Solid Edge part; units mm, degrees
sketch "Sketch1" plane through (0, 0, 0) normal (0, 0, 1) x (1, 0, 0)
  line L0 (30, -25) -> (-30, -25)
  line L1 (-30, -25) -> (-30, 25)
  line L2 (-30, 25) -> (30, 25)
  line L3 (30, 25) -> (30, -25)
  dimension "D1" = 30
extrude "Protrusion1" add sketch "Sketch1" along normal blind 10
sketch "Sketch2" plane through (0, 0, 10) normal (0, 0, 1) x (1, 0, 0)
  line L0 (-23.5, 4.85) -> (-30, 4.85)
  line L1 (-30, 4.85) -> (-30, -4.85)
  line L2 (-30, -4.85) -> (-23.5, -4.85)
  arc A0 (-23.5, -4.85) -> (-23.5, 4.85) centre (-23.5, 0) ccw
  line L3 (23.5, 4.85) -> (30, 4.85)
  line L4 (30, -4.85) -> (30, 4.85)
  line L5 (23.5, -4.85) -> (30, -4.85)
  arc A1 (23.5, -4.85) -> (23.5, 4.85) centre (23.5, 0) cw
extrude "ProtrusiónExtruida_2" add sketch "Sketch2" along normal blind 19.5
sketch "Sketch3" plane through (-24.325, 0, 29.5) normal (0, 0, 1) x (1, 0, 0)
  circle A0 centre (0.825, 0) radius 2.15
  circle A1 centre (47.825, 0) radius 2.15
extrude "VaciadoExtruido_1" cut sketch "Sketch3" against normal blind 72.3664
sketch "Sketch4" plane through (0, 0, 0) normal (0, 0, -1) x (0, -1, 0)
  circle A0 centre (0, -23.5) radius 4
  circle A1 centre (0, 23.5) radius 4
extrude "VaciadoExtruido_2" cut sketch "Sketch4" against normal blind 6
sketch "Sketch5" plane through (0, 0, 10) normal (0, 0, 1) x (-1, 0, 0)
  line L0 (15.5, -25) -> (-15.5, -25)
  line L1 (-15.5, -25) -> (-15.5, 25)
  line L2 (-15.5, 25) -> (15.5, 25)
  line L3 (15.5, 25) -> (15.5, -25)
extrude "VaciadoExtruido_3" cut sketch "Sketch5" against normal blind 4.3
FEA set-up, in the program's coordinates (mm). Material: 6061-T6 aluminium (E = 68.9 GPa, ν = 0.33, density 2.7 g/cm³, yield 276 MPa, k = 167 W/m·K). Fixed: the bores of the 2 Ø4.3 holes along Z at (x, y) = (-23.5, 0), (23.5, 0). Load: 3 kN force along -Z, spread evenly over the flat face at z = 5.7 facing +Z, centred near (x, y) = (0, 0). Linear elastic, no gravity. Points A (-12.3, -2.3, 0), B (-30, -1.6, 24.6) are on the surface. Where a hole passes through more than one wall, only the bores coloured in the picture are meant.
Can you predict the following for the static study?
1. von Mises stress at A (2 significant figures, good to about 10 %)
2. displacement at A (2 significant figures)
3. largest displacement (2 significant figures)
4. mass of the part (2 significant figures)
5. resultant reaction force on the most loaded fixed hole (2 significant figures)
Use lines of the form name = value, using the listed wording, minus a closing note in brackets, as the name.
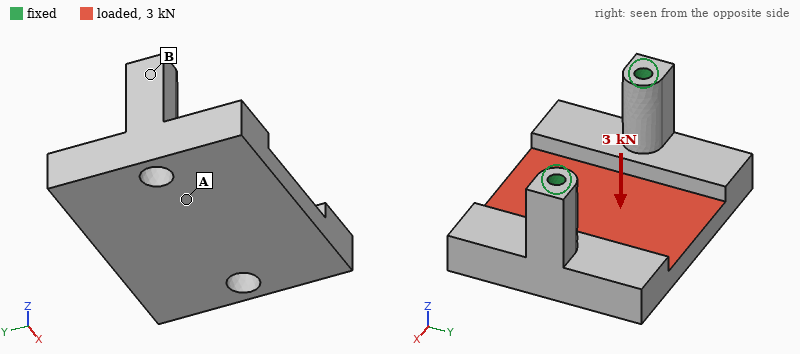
von Mises stress at A = 25 MPa
displacement at A = 13 µm
largest displacement = 39 µm
mass of the part = 70 g
resultant reaction force on the most loaded fixed hole = 2.2 kN
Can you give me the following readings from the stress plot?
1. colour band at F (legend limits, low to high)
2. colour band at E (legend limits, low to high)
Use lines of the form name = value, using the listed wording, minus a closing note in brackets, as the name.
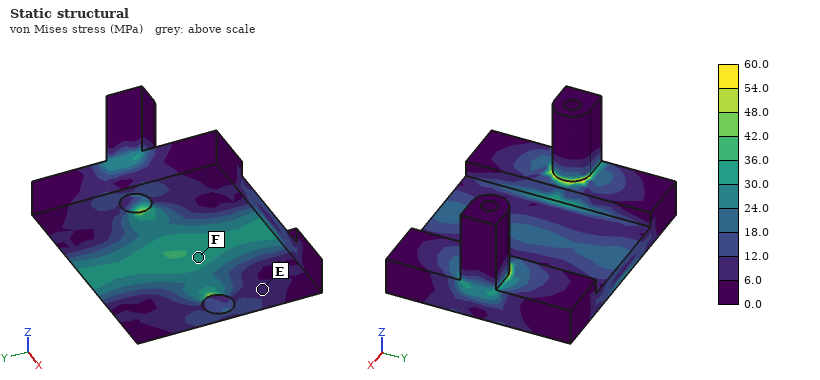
colour band at F = 30.0 to 36.0 MPa
colour band at E = 6.0 to 12.0 MPa
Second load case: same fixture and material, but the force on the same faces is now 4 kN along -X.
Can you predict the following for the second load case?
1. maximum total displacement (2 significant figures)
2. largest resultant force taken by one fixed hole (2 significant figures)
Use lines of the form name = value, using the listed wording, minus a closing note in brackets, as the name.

maximum total displacement = 11 µm
largest resultant force taken by one fixed hole = 2.0 kN
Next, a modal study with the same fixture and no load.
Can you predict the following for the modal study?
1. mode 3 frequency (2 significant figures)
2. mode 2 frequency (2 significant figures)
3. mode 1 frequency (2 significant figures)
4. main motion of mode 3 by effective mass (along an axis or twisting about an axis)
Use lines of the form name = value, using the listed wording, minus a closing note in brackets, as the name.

mode 3 frequency = 9600 Hz
mode 2 frequency = 8500 Hz
mode 1 frequency = 5200 Hz
main motion of mode 3 by effective mass = along Z
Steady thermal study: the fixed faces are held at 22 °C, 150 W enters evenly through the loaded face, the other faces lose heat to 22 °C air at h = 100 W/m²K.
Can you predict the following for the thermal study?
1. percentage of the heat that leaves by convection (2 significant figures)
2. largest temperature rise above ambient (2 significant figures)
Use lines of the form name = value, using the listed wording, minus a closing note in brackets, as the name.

percentage of the heat that leaves by convection = 11 %
largest temperature rise above ambient = 40 K
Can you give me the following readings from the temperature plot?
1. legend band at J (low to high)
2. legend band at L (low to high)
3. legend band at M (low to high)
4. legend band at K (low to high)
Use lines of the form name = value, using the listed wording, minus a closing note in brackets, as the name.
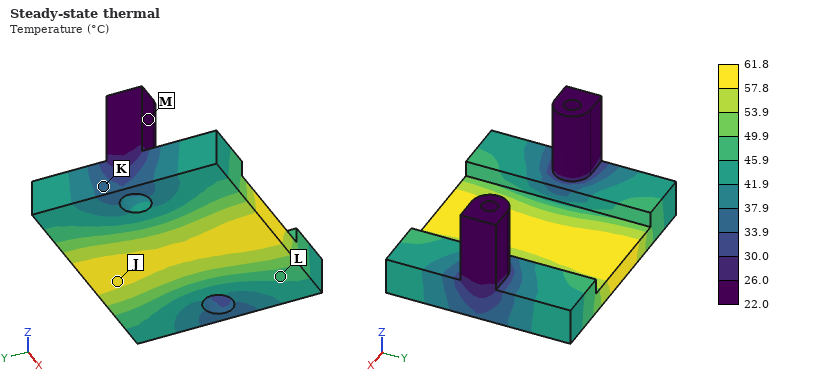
legend band at J = 57.8 to 61.8 °C
legend band at L = 45.9 to 49.9 °C
legend band at M = 22.0 to 26.0 °C
legend band at K = 33.9 to 37.9 °C
